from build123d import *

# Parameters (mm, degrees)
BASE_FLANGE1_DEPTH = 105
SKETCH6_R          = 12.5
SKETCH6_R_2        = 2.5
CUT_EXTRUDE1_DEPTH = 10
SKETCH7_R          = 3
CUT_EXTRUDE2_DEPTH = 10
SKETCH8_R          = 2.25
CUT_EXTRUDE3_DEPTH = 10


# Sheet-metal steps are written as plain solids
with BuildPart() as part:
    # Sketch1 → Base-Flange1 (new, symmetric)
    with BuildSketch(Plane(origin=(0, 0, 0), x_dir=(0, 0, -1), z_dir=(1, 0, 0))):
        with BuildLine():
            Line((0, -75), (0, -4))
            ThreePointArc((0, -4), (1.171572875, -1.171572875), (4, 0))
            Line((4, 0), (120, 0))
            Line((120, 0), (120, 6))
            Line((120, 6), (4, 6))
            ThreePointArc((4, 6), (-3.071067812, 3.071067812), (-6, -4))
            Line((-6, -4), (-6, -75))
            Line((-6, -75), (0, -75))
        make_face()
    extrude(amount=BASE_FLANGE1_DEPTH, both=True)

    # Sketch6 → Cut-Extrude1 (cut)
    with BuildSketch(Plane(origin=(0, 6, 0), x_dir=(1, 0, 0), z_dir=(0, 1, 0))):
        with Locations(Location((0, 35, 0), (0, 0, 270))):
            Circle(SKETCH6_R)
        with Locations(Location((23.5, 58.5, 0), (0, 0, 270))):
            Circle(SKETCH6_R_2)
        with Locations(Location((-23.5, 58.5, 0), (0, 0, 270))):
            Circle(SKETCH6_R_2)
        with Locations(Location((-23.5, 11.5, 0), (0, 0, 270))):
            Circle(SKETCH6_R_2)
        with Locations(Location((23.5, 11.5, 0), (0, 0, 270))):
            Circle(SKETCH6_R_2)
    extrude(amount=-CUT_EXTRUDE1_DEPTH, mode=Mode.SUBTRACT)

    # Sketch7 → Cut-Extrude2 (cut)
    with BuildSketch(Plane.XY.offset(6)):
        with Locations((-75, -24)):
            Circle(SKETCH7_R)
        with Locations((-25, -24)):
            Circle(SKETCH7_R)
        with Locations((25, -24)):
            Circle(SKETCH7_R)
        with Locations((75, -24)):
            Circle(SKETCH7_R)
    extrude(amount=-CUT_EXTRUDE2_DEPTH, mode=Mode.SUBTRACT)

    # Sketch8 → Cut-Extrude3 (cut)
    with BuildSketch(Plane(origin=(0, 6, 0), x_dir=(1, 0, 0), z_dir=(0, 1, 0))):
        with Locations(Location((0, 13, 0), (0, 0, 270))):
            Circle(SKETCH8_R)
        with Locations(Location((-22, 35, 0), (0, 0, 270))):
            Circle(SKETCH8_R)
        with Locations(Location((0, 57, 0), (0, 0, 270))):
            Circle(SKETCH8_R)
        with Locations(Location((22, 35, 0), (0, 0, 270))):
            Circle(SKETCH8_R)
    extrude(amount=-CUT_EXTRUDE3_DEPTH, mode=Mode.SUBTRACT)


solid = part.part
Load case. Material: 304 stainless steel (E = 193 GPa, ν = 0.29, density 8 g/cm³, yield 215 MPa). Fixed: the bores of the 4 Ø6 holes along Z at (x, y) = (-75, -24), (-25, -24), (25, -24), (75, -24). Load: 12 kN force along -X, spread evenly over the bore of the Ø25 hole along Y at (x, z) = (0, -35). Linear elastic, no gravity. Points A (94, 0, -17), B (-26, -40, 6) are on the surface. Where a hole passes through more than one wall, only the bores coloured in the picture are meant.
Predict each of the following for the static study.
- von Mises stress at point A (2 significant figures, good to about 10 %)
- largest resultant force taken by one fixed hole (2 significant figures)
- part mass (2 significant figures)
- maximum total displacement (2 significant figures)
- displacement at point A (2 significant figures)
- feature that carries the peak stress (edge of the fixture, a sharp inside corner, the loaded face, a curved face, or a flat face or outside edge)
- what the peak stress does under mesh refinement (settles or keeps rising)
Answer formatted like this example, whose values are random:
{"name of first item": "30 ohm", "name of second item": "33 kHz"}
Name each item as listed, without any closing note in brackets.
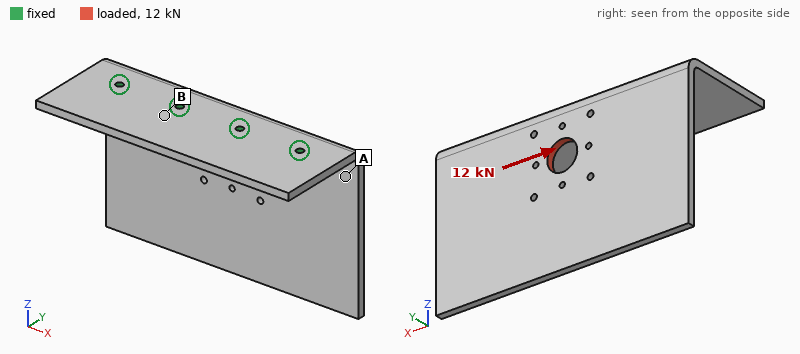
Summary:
{"von Mises stress at point A": "42 MPa", "largest resultant force taken by one fixed hole": "4.3 kN", "part mass": "2.0 kg", "maximum total displacement": "0.30 mm", "displacement at point A": "0.12 mm", "feature that carries the peak stress": "edge of the fixture", "what the peak stress does under mesh refinement": "keeps rising"}
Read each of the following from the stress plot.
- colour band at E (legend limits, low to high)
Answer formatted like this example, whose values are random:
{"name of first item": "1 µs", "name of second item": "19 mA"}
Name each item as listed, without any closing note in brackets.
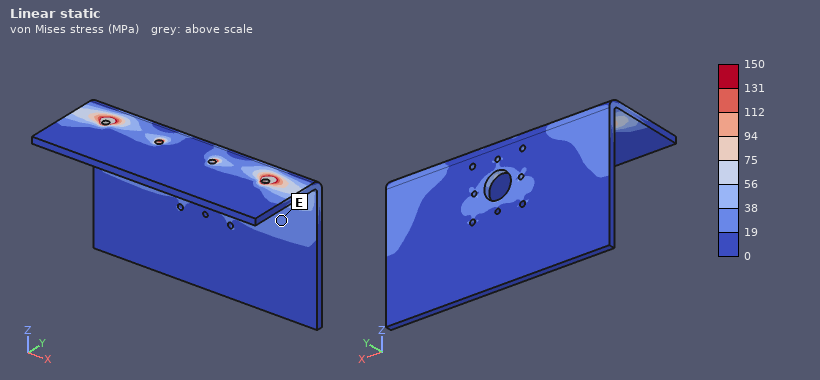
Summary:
{"colour band at E": "19 to 38 MPa"}
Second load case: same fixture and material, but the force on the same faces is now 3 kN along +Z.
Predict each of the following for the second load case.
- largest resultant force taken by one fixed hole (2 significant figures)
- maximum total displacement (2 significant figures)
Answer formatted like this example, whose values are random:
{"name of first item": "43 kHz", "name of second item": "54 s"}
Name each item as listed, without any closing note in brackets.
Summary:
{"largest resultant force taken by one fixed hole": "790 N", "maximum total displacement": "0.23 mm"}
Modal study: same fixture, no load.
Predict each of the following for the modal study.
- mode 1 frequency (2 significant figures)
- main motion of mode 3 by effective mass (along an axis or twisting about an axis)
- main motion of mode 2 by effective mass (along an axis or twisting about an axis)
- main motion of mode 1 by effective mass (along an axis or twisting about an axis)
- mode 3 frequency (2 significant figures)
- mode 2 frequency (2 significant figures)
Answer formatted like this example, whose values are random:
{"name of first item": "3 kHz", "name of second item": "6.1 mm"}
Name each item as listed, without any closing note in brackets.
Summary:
{"mode 1 frequency": "230 Hz", "main motion of mode 3 by effective mass": "along X", "main motion of mode 2 by effective mass": "twisting about Z", "main motion of mode 1 by effective mass": "along Y", "mode 3 frequency": "1000 Hz", "mode 2 frequency": "440 Hz"}
